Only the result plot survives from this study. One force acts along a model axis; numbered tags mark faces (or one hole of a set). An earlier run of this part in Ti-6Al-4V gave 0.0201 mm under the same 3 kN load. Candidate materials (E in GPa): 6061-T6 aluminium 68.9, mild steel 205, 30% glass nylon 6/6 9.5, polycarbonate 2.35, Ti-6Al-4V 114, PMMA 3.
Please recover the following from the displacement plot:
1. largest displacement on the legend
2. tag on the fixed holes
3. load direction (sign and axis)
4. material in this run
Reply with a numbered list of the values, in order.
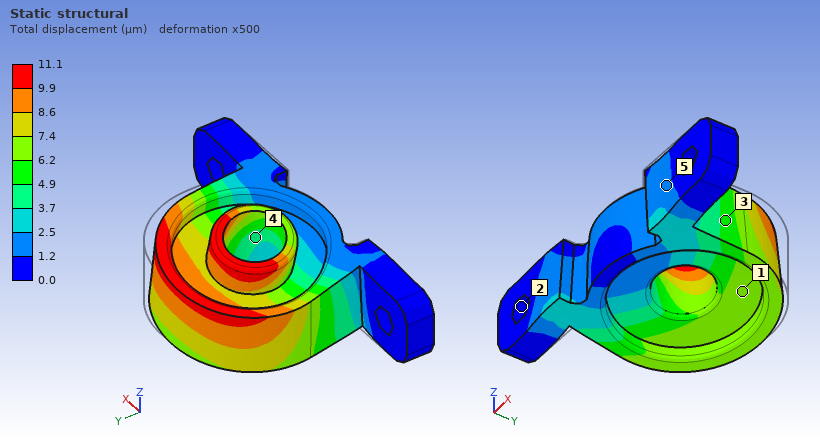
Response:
1. 11.1 µm
2. 2
3. -X
4. mild steel
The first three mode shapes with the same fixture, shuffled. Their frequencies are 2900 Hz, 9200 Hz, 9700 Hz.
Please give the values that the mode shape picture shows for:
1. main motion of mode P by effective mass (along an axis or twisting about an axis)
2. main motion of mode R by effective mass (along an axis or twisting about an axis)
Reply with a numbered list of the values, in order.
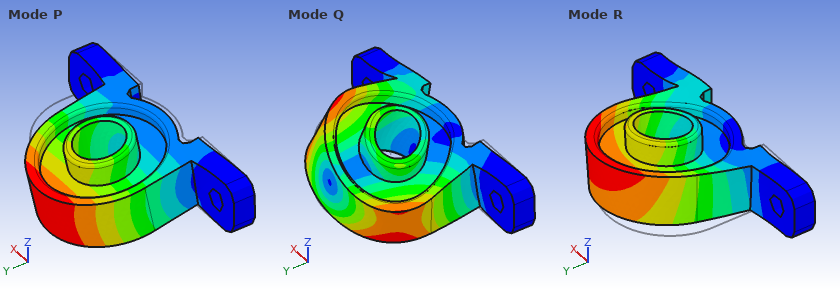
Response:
1. along Z
2. along X
